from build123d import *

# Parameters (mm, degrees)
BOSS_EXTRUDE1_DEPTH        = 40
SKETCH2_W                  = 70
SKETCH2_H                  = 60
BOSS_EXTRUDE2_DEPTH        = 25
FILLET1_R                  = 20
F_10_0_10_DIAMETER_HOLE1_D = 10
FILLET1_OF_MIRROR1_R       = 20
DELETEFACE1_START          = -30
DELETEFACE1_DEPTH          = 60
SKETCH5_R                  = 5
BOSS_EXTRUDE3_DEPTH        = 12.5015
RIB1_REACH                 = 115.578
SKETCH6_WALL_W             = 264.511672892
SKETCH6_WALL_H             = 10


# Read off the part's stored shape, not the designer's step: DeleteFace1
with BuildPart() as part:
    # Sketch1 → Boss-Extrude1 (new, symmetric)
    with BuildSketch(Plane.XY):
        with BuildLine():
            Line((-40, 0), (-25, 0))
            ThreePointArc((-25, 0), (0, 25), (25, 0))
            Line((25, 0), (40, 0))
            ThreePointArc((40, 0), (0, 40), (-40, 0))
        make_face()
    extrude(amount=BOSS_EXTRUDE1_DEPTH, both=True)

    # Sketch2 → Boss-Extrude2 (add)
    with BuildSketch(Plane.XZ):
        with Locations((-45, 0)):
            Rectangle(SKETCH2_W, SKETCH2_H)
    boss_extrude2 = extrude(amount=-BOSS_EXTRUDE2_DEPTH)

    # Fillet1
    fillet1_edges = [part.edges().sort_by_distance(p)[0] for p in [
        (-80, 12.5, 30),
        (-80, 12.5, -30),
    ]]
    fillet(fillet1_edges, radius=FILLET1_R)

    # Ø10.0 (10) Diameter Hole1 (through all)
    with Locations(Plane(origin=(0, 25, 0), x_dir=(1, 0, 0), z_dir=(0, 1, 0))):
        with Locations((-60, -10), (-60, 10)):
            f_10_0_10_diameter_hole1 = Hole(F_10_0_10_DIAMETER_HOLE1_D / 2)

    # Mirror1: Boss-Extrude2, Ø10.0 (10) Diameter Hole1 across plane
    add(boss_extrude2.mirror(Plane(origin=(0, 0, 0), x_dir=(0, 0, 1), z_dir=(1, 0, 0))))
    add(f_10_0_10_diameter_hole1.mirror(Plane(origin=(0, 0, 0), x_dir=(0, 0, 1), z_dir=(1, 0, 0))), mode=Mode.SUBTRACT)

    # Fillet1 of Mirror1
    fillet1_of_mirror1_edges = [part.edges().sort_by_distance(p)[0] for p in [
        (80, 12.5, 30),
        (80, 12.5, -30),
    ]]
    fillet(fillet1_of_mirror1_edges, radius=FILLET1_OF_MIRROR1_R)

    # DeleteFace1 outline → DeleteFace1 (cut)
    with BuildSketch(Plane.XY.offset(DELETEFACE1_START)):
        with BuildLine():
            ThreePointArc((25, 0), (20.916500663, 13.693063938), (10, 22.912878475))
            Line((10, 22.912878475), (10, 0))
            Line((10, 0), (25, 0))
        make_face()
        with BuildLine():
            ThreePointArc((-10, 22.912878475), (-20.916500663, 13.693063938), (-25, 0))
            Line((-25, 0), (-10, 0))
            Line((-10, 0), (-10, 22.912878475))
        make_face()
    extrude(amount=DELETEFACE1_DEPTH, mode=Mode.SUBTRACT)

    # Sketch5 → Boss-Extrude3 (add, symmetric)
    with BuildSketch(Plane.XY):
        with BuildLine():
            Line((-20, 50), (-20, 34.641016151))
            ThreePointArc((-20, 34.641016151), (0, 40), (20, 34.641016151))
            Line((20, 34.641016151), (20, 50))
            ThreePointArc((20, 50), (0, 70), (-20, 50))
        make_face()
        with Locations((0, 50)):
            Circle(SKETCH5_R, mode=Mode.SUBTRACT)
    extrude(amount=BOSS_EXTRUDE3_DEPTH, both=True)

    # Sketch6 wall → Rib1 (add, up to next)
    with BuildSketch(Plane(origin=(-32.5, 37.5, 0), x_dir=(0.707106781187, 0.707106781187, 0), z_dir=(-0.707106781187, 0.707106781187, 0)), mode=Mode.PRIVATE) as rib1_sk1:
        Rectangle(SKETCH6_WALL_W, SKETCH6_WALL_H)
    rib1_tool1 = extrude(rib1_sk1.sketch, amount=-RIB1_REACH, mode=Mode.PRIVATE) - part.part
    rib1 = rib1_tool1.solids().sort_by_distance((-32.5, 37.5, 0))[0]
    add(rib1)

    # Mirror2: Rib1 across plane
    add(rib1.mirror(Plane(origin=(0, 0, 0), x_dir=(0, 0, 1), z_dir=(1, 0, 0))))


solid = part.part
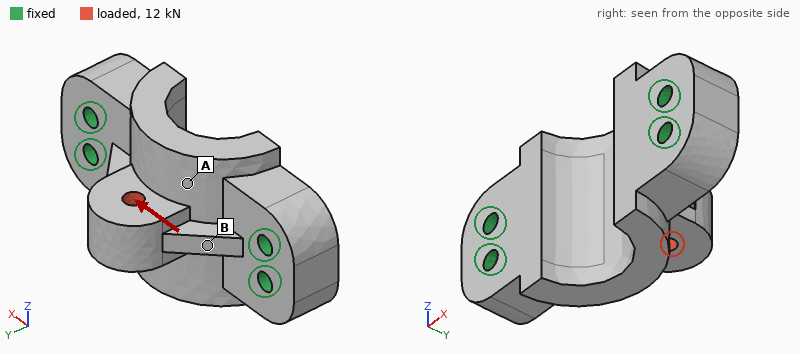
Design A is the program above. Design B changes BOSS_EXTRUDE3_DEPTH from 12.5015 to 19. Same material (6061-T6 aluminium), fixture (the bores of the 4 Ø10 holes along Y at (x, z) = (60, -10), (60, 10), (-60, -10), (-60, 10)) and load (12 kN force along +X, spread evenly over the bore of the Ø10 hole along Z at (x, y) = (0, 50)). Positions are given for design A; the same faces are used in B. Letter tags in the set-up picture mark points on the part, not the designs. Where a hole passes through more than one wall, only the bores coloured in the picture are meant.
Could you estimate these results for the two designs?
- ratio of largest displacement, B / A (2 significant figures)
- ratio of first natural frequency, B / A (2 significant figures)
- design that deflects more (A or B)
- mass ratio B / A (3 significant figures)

0.89
0.92
A
1.05
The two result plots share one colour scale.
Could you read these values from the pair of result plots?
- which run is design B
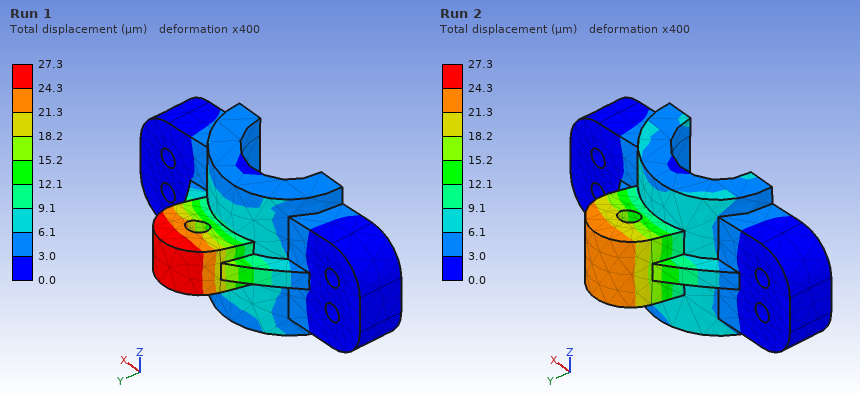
Run 2
